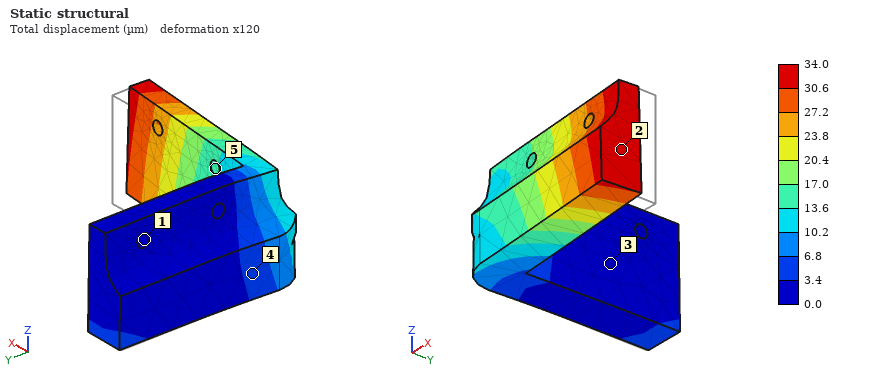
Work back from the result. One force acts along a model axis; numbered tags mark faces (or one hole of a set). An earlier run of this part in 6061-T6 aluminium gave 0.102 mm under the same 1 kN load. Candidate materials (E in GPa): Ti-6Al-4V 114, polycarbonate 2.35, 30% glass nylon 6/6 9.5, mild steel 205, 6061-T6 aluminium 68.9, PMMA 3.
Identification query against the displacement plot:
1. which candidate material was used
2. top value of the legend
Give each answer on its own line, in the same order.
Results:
mild steel
34.0 µm
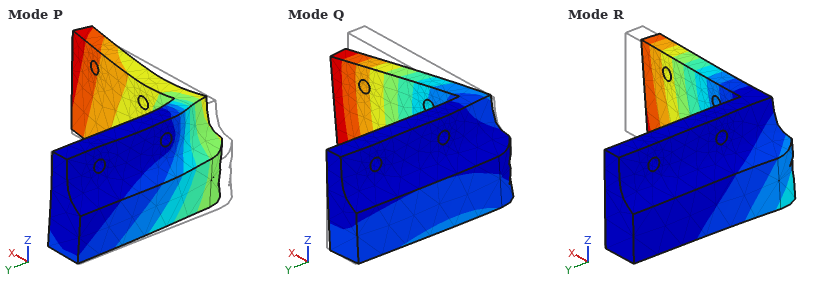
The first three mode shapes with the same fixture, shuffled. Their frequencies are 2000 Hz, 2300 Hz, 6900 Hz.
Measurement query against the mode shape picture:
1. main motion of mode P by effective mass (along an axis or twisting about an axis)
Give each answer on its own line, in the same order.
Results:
along X
